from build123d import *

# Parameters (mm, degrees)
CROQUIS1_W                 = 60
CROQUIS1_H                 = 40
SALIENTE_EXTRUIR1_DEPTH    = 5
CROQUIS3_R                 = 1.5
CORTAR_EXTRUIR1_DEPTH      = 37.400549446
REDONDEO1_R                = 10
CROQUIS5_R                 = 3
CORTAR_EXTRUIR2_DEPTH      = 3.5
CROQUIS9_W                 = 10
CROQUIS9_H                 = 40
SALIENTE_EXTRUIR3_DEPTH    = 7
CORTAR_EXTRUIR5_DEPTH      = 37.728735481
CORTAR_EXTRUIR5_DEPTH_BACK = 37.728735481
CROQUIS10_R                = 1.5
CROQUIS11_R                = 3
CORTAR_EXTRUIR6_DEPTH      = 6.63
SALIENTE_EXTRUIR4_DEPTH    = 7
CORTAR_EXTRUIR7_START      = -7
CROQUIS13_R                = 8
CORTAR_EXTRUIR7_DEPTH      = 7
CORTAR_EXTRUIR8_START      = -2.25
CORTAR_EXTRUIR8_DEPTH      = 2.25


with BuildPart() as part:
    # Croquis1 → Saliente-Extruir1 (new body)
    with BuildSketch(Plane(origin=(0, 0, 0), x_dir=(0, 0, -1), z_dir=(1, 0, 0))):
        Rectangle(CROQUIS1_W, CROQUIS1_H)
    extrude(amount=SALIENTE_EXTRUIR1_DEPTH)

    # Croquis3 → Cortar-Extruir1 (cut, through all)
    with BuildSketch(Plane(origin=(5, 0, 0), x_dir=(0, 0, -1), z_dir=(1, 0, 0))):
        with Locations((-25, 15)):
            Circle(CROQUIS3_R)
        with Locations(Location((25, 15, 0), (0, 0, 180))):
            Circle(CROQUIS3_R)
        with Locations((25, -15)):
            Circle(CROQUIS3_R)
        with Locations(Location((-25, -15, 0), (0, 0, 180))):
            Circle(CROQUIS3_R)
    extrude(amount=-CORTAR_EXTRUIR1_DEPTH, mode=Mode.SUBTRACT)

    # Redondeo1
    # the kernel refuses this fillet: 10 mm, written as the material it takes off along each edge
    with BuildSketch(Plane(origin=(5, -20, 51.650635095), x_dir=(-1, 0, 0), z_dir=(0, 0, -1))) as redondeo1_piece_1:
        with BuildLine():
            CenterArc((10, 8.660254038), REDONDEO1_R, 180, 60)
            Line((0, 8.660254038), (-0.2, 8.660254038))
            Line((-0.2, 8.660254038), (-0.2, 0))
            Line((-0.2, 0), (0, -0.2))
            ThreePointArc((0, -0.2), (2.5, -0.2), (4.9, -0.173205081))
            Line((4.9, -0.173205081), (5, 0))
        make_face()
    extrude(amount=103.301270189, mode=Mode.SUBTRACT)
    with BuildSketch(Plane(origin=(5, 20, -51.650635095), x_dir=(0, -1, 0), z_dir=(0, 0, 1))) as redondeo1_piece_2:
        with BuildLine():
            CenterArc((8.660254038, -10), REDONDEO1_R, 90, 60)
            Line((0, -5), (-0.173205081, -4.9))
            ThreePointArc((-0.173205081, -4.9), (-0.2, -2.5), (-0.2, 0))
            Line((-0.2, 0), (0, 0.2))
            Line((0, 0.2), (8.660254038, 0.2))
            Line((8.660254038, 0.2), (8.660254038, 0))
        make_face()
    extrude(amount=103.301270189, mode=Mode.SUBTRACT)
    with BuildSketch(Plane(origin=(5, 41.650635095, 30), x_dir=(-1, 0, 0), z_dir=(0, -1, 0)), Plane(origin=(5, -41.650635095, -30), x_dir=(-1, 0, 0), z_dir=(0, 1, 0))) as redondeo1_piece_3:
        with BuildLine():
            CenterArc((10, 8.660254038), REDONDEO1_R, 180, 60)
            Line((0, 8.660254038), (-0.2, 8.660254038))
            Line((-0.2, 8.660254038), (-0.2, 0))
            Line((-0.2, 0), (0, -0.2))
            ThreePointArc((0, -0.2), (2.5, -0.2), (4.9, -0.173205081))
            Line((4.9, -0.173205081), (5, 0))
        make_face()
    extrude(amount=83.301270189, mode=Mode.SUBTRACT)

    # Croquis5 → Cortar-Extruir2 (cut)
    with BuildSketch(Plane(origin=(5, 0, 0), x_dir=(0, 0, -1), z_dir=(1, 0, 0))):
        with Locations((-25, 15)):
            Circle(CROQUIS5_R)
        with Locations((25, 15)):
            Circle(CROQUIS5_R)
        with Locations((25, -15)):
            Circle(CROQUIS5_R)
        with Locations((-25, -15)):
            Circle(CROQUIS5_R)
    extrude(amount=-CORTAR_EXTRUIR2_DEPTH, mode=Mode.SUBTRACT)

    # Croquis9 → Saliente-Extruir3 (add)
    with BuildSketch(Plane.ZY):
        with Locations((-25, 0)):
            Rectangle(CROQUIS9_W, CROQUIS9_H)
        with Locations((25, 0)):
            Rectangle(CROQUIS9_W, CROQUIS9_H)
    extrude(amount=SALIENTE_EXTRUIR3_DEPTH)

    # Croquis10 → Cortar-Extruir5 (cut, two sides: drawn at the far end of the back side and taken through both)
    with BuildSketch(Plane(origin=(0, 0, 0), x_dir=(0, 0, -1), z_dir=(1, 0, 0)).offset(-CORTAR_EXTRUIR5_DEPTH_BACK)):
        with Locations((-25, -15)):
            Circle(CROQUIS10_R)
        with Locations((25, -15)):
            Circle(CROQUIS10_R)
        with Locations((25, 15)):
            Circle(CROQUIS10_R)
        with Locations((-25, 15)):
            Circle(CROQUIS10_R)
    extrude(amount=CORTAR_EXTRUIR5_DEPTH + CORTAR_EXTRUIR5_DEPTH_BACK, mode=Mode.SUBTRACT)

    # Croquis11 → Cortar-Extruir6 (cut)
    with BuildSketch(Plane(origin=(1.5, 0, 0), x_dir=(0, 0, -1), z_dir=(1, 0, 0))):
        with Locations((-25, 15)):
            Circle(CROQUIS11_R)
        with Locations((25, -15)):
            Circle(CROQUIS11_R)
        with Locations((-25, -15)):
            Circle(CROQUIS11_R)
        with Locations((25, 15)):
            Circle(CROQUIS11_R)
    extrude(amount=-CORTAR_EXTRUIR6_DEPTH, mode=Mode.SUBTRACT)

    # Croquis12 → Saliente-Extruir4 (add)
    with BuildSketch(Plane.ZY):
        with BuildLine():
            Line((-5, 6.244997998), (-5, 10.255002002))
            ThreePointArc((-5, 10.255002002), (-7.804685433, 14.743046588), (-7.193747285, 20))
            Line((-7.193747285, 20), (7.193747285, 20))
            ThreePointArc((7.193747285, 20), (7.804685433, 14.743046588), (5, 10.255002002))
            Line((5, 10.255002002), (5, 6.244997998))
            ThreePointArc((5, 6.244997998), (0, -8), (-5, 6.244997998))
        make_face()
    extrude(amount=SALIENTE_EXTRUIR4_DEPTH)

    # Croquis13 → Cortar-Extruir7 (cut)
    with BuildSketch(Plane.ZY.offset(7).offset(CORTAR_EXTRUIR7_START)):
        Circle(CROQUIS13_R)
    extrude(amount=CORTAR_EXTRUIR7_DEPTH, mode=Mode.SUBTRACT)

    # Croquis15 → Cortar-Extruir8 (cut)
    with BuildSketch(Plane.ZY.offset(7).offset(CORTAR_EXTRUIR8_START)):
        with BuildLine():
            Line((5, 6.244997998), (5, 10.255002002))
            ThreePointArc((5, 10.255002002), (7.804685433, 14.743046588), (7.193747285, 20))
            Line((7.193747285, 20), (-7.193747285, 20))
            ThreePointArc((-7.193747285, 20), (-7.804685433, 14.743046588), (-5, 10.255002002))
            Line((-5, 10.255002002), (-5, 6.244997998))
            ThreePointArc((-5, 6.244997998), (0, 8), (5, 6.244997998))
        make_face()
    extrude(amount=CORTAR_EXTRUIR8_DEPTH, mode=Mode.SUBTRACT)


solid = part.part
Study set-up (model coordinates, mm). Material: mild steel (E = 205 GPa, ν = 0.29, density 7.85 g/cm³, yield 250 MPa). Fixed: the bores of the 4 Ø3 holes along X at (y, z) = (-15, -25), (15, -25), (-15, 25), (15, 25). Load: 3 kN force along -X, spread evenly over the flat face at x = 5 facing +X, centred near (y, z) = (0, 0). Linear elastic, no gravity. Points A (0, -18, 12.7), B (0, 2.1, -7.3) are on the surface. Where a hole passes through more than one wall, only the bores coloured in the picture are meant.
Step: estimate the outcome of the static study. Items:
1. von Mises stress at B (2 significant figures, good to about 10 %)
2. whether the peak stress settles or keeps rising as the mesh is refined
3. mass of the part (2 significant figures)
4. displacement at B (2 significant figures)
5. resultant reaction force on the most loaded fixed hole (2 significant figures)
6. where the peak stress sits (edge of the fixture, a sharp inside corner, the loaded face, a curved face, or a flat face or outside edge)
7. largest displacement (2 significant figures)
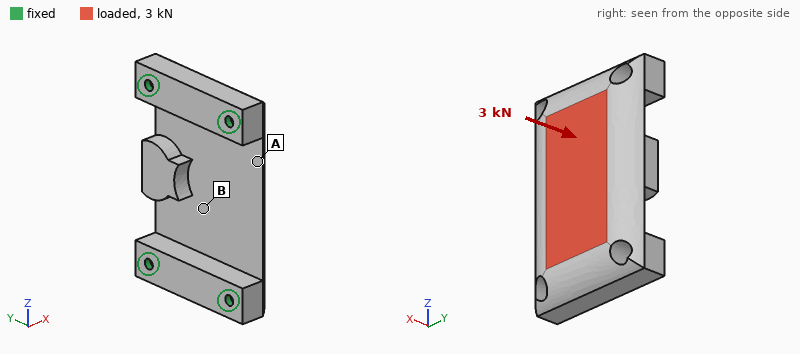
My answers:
27 MPa
keeps rising
120 g
15 µm
1.1 kN
edge of the fixture
17 µm
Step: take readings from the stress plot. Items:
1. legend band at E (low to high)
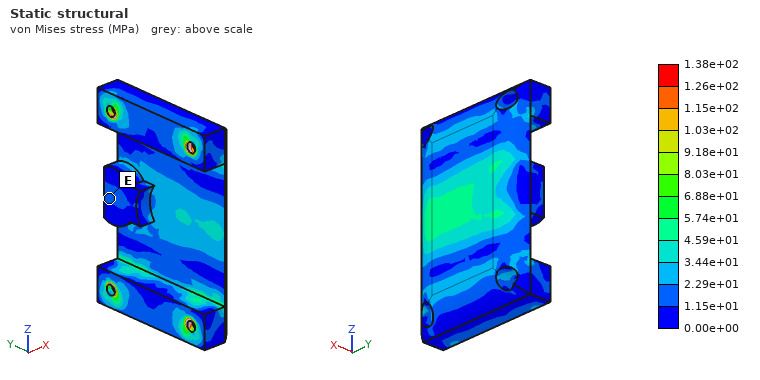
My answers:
1.15e+01 to 2.29e+01 MPa
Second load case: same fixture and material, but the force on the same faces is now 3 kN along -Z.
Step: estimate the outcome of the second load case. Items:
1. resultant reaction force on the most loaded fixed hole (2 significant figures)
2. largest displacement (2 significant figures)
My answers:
810 N
12 µm
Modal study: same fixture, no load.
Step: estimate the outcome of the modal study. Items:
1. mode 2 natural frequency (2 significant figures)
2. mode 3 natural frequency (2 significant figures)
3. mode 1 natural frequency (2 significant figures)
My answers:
9000 Hz
12 kHz
9000 Hz
